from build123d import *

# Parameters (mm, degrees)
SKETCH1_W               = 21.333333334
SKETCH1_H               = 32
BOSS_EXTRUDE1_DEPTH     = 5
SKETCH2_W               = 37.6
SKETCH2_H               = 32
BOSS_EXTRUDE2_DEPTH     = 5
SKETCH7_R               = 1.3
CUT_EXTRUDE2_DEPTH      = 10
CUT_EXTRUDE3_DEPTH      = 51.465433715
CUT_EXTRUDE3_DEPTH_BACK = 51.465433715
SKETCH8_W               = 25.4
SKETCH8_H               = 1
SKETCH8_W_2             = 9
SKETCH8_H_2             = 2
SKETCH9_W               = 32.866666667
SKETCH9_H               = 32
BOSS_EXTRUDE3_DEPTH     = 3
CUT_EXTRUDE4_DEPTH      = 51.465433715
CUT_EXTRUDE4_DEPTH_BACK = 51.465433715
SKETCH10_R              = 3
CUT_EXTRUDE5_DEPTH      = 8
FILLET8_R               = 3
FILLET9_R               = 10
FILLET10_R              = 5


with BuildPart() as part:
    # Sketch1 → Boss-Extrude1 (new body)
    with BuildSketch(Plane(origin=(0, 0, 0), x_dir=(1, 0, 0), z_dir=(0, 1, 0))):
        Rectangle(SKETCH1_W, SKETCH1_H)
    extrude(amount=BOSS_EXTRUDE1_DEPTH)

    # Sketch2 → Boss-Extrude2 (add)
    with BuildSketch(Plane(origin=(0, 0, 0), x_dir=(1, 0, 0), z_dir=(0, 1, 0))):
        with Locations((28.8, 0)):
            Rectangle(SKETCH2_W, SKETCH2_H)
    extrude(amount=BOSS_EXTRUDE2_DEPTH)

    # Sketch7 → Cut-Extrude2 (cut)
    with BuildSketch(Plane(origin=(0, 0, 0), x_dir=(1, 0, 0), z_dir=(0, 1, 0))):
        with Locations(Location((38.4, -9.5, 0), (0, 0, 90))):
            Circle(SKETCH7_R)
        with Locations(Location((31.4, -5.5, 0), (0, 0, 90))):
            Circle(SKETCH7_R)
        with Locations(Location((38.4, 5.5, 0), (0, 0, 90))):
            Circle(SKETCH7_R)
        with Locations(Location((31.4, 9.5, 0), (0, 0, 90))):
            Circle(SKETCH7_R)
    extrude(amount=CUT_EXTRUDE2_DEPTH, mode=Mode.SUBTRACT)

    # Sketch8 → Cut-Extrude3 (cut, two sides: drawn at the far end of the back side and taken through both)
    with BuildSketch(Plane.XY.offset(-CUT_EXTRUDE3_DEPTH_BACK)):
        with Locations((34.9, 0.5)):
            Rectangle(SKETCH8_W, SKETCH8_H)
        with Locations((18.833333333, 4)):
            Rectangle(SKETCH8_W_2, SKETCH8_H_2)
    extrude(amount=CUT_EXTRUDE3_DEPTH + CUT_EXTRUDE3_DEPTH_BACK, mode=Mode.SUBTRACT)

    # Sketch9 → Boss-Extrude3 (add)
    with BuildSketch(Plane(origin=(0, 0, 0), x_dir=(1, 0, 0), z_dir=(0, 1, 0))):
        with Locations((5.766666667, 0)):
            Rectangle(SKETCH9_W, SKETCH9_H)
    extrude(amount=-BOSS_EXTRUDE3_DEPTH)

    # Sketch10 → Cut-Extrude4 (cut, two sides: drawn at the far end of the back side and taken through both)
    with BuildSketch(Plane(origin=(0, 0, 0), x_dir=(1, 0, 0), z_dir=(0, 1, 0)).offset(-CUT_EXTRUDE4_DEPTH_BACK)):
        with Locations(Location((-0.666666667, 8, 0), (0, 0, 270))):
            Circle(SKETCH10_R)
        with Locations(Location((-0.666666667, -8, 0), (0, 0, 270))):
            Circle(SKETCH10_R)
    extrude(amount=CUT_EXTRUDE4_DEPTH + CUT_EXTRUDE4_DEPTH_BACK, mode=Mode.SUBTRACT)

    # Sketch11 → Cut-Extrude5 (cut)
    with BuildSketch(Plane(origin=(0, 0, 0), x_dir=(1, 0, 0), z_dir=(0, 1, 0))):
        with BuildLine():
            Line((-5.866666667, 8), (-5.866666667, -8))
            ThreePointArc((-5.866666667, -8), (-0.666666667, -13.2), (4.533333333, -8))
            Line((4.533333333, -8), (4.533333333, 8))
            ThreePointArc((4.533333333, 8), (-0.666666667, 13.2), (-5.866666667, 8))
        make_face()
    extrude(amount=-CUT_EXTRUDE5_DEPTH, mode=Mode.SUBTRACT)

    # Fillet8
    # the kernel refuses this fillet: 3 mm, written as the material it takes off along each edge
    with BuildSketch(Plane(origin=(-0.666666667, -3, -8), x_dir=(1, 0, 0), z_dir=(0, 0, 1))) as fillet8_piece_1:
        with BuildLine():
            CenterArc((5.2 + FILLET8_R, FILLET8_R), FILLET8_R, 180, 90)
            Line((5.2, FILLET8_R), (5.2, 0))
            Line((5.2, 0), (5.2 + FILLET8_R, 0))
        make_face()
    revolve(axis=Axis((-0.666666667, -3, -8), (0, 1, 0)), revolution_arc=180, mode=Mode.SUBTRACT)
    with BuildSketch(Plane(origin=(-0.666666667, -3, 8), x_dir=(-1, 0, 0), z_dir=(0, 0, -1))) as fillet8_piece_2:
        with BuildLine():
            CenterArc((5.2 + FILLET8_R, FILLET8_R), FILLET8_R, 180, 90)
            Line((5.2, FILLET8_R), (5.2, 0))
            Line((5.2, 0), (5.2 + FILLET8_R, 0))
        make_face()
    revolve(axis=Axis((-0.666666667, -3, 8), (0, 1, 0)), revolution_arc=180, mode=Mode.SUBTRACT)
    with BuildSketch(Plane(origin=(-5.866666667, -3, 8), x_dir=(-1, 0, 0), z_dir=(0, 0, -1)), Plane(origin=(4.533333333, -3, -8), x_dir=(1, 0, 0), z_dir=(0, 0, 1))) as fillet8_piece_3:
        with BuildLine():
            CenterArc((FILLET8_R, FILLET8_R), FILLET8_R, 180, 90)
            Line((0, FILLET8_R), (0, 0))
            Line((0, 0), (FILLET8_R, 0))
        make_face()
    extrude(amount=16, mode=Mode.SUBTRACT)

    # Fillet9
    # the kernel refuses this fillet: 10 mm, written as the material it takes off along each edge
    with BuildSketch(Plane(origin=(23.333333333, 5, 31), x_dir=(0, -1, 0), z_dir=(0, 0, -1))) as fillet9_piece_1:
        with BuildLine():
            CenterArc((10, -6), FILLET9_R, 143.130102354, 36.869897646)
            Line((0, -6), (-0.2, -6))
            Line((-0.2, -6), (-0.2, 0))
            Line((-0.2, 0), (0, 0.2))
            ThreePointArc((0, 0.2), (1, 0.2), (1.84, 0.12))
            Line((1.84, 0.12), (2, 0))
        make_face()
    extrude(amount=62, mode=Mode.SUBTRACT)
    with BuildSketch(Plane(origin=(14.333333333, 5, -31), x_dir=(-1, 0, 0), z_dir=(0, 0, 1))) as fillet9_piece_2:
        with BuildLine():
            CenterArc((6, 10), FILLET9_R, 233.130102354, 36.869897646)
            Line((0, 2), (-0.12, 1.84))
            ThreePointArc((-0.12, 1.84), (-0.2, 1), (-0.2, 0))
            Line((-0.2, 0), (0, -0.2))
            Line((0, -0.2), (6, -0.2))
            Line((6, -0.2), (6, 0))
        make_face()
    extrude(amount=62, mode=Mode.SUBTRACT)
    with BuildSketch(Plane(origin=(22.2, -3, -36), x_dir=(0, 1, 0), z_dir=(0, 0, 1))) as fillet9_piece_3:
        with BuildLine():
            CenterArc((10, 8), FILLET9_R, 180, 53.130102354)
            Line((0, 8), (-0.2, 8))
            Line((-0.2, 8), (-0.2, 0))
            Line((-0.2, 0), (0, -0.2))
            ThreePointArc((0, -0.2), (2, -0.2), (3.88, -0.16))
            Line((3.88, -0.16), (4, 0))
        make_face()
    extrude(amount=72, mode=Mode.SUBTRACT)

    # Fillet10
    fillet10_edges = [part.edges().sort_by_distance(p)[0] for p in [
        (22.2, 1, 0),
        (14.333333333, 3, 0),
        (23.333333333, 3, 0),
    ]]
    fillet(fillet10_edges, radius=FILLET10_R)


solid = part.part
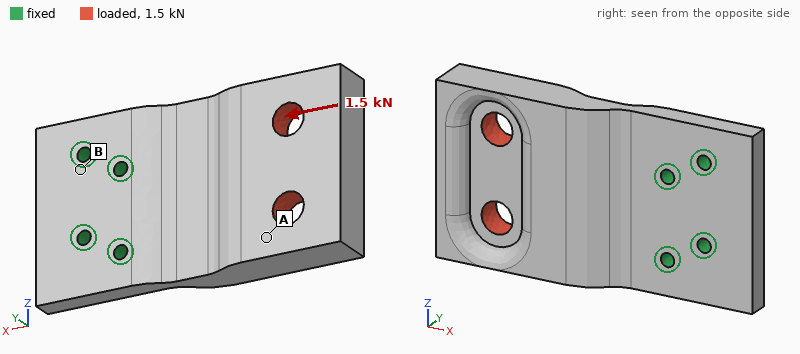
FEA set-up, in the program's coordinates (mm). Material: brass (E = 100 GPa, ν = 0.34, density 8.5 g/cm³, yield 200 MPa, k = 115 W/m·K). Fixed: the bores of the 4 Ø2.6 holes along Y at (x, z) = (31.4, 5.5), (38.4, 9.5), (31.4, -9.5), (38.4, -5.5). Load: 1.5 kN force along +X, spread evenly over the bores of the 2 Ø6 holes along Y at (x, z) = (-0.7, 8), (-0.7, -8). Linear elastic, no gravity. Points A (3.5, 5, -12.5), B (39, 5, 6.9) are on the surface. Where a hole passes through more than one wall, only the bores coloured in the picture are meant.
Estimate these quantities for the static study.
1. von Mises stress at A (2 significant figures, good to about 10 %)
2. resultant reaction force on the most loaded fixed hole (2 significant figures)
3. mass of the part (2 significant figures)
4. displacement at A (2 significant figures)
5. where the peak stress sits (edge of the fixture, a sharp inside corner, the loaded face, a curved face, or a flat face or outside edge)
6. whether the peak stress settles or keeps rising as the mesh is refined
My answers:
12 MPa
540 N
79 g
21 µm
edge of the fixture
keeps rising
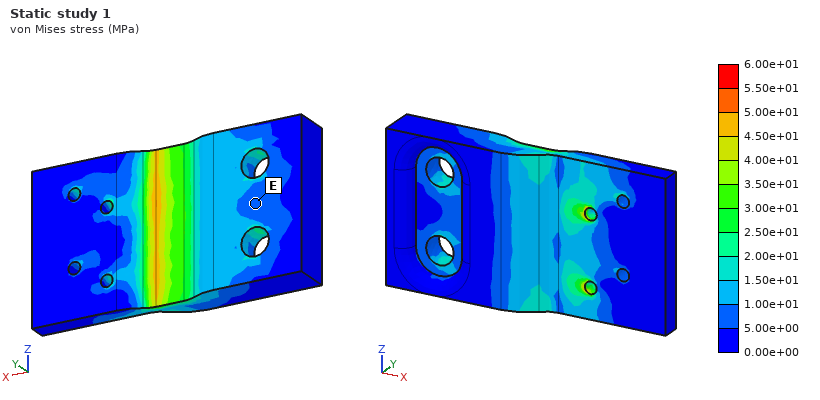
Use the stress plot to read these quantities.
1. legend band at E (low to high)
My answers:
5.00e+00 to 1.00e+01 MPa
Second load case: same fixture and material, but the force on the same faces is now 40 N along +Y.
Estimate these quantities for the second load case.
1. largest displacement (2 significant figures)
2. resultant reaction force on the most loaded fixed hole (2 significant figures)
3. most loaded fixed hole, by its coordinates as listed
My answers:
59 µm
66 N
(31.4, 5.5)
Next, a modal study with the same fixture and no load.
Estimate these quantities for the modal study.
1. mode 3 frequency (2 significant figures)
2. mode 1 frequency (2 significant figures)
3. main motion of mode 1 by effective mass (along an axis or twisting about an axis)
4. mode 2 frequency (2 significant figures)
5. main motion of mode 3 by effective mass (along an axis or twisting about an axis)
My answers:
4900 Hz
780 Hz
along Y
3300 Hz
along Z
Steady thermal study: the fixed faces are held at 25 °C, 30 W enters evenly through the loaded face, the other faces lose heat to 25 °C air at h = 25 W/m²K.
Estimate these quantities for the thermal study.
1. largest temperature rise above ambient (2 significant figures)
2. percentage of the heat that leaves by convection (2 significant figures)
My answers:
60 K
12 %
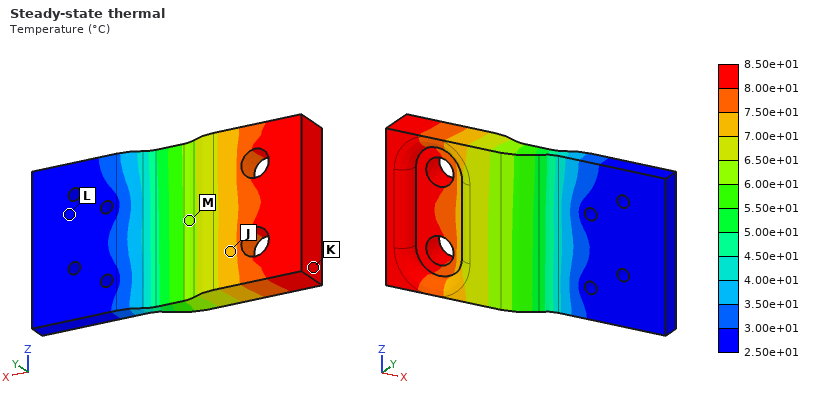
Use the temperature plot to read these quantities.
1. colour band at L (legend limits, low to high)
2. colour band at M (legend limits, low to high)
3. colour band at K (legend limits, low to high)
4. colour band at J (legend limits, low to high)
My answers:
2.50e+01 to 3.00e+01 °C
6.00e+01 to 6.50e+01 °C
8.00e+01 to 8.50e+01 °C
7.00e+01 to 7.50e+01 °C
